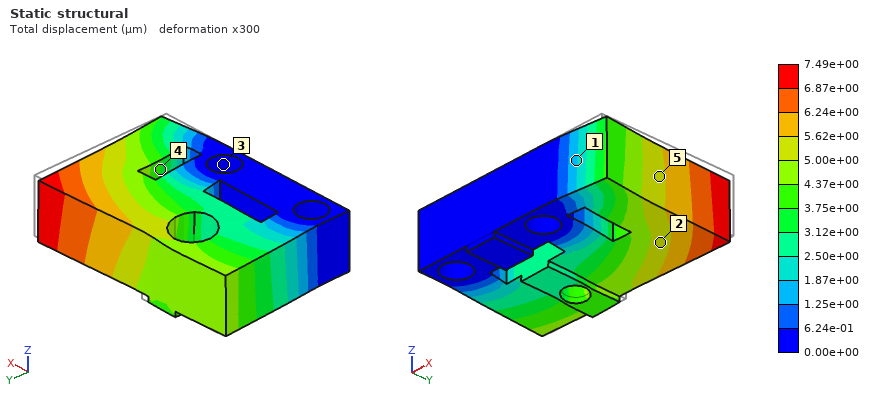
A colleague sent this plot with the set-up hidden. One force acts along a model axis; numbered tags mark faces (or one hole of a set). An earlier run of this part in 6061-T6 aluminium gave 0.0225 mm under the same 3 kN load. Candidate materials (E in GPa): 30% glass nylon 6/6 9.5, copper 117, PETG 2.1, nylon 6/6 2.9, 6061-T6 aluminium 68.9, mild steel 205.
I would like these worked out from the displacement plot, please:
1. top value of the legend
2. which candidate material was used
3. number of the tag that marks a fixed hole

7.49e+00 µm
mild steel
3
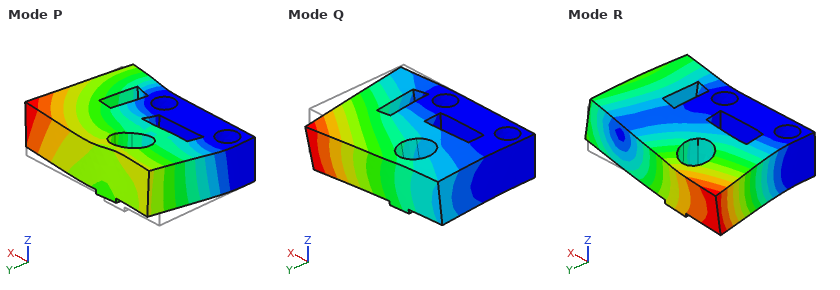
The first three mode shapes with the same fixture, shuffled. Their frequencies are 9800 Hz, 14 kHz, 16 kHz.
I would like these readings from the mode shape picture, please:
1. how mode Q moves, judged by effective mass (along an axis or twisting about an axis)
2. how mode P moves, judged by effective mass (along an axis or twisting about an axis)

along Z
along X
